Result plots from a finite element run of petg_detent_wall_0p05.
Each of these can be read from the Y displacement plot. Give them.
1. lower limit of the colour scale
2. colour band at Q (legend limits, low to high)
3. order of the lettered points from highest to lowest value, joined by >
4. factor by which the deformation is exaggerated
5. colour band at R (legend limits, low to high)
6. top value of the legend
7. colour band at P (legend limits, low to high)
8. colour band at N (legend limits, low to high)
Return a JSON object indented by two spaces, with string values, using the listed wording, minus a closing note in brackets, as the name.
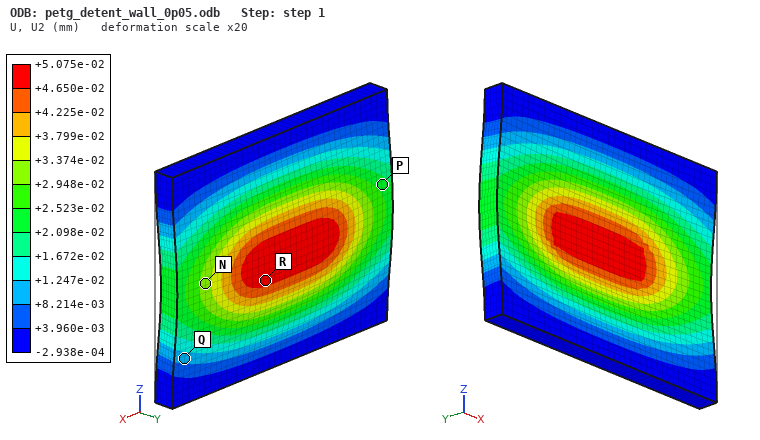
{
  "lower limit of the colour scale": "-2.938e-04 mm",
  "colour band at Q": "+8.214e-03 to +1.247e-02 mm",
  "order of the lettered points from highest to lowest value, joined by >": "R > N > P > Q",
  "factor by which the deformation is exaggerated": "20",
  "colour band at R": "+4.650e-02 to +5.075e-02 mm",
  "top value of the legend": "+5.075e-02 mm",
  "colour band at P": "+2.098e-02 to +2.523e-02 mm",
  "colour band at N": "+2.948e-02 to +3.374e-02 mm"
}
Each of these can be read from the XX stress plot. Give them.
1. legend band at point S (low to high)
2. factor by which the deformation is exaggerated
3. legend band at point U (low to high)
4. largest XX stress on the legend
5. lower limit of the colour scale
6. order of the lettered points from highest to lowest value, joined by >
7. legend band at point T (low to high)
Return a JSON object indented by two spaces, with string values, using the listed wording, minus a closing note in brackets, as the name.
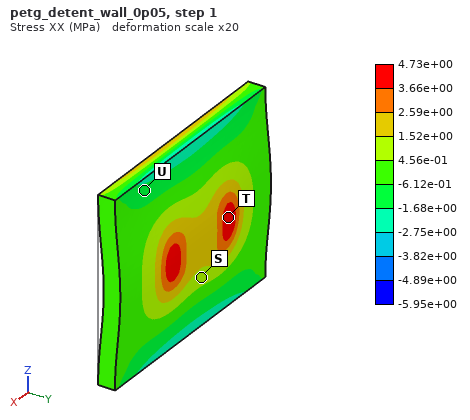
{
  "legend band at point S": "4.56e-01 to 1.52e+00 MPa",
  "factor by which the deformation is exaggerated": "20",
  "legend band at point U": "-1.68e+00 to -6.12e-01 MPa",
  "largest XX stress on the legend": "4.73e+00 MPa",
  "lower limit of the colour scale": "-5.95e+00 MPa",
  "order of the lettered points from highest to lowest value, joined by >": "T > S > U",
  "legend band at point T": "3.66e+00 to 4.73e+00 MPa"
}
